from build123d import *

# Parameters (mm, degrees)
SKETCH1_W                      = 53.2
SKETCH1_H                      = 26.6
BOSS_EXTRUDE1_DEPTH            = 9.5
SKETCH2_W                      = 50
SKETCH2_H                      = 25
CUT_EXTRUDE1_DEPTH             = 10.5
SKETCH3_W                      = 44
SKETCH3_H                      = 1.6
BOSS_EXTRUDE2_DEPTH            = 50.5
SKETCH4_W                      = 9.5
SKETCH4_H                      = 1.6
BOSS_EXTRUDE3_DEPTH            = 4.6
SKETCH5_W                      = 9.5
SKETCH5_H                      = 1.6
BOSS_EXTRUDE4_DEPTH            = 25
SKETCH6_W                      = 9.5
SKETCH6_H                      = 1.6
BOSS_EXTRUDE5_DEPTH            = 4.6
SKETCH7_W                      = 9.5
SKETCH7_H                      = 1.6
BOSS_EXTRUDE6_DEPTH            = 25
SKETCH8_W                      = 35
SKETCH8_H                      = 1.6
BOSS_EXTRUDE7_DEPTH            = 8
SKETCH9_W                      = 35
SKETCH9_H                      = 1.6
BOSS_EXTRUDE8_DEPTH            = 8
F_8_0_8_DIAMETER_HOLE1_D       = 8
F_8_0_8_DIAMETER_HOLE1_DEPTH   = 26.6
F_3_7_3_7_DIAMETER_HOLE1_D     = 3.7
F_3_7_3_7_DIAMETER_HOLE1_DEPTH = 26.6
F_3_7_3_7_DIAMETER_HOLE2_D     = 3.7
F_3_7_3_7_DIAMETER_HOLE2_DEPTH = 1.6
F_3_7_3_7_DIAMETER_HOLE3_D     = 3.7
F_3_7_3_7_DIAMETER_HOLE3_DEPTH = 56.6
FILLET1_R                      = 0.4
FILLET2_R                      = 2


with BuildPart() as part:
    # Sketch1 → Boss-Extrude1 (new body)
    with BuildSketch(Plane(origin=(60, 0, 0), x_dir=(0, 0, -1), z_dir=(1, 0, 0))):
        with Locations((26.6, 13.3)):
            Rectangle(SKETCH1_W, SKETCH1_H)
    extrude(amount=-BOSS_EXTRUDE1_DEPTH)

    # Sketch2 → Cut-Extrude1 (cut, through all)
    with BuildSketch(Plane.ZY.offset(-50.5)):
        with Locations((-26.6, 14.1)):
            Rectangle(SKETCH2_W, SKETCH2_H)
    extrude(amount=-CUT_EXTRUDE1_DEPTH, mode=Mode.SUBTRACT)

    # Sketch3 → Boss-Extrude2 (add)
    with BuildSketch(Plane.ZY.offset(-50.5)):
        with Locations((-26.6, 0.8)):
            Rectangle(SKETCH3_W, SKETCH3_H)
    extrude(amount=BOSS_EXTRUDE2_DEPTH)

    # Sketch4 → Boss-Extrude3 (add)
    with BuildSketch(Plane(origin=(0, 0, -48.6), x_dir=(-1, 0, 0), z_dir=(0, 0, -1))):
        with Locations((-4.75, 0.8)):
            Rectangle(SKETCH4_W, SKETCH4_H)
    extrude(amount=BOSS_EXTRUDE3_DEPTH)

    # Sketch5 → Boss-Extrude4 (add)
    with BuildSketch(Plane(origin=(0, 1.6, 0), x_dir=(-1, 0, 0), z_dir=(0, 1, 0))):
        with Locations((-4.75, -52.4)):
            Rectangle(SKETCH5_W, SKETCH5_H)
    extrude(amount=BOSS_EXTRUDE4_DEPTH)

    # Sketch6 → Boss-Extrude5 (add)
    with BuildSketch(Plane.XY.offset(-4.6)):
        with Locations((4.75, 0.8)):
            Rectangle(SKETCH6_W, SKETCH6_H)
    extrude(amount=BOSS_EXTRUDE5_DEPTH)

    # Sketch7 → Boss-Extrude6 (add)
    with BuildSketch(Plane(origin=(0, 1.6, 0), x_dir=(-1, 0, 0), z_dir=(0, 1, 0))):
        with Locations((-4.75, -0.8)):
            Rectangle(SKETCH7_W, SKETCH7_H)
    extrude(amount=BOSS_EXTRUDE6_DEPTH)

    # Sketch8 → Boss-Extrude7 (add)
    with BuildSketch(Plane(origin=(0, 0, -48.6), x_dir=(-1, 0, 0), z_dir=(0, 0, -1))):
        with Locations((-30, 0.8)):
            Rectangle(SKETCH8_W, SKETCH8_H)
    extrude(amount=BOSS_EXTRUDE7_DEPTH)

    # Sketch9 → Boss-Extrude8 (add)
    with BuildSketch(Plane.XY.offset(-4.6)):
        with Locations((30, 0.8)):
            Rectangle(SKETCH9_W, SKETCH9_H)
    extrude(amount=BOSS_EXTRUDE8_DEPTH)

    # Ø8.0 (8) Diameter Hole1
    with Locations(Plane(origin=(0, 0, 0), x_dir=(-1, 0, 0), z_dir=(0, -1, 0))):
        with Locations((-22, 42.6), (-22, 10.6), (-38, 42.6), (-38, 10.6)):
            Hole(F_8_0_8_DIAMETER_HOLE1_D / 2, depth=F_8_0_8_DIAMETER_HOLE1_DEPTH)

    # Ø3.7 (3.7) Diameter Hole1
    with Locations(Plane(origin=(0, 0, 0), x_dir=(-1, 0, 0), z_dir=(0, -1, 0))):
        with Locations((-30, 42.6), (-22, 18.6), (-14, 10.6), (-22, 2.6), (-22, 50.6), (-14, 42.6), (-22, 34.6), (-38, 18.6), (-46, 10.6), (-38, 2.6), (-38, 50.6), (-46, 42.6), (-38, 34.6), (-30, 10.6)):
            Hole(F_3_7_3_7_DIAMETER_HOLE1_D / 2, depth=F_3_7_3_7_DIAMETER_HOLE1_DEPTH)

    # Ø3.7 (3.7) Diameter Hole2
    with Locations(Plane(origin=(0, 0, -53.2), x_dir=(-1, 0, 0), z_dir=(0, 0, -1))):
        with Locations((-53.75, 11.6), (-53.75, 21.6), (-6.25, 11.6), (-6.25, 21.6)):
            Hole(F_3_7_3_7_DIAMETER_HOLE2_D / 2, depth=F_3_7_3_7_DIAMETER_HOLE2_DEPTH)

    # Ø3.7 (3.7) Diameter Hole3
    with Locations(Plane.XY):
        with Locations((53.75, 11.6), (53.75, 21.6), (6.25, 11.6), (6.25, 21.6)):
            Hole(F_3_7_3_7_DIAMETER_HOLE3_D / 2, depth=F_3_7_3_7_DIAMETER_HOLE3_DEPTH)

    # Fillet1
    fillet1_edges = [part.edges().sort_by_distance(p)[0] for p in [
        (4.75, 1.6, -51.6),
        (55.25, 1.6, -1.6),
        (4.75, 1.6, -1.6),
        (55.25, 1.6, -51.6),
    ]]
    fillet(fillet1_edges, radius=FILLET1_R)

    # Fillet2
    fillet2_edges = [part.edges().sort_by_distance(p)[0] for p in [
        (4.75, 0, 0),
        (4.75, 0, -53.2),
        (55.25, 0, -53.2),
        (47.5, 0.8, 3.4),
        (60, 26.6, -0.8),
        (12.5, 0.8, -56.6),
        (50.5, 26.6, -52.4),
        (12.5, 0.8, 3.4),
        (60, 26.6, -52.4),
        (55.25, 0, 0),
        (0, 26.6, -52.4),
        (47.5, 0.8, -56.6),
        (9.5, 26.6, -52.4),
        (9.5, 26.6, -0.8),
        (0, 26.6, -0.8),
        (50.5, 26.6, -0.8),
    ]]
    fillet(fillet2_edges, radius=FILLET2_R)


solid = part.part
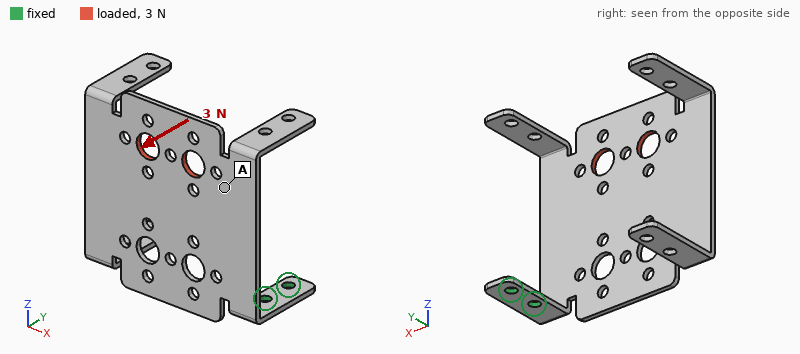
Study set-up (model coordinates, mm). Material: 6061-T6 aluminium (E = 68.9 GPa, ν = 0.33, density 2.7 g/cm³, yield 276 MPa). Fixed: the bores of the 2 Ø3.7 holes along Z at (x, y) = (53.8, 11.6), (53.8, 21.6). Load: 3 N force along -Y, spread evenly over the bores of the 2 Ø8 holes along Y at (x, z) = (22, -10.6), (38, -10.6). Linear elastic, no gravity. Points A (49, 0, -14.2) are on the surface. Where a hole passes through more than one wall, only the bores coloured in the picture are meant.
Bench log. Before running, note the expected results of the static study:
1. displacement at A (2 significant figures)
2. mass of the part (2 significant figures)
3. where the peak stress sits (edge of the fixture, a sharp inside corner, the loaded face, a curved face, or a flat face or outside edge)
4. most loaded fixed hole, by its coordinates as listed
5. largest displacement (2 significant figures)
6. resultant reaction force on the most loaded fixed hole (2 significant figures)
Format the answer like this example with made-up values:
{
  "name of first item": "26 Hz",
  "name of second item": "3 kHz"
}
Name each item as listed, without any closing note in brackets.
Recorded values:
{
  "displacement at A": "0.40 mm",
  "mass of the part": "17 g",
  "where the peak stress sits": "a curved face",
  "most loaded fixed hole, by its coordinates as listed": "(53.8, 11.6)",
  "largest displacement": "0.82 mm",
  "resultant reaction force on the most loaded fixed hole": "6.6 N"
}
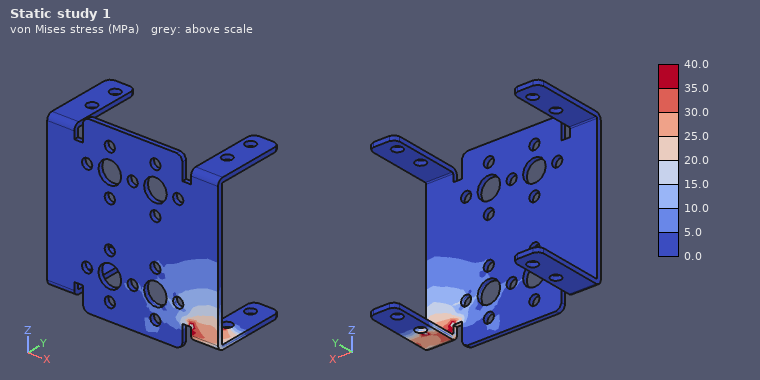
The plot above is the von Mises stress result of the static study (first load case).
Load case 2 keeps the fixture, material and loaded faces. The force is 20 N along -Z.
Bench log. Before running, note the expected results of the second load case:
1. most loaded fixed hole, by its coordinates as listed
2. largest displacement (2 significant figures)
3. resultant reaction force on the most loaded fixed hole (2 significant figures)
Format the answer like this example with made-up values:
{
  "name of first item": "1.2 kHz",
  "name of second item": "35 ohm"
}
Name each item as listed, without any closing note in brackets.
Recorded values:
{
  "most loaded fixed hole, by its coordinates as listed": "(53.8, 11.6)",
  "largest displacement": "1.0 mm",
  "resultant reaction force on the most loaded fixed hole": "15 N"
}
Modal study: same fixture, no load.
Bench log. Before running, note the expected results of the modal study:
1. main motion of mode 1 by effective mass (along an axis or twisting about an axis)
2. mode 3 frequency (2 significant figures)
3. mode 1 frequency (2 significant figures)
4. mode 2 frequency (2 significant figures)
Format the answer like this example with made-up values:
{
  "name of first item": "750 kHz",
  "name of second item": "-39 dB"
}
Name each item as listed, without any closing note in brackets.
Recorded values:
{
  "main motion of mode 1 by effective mass": "along Y",
  "mode 3 frequency": "250 Hz",
  "mode 1 frequency": "120 Hz",
  "mode 2 frequency": "170 Hz"
}
